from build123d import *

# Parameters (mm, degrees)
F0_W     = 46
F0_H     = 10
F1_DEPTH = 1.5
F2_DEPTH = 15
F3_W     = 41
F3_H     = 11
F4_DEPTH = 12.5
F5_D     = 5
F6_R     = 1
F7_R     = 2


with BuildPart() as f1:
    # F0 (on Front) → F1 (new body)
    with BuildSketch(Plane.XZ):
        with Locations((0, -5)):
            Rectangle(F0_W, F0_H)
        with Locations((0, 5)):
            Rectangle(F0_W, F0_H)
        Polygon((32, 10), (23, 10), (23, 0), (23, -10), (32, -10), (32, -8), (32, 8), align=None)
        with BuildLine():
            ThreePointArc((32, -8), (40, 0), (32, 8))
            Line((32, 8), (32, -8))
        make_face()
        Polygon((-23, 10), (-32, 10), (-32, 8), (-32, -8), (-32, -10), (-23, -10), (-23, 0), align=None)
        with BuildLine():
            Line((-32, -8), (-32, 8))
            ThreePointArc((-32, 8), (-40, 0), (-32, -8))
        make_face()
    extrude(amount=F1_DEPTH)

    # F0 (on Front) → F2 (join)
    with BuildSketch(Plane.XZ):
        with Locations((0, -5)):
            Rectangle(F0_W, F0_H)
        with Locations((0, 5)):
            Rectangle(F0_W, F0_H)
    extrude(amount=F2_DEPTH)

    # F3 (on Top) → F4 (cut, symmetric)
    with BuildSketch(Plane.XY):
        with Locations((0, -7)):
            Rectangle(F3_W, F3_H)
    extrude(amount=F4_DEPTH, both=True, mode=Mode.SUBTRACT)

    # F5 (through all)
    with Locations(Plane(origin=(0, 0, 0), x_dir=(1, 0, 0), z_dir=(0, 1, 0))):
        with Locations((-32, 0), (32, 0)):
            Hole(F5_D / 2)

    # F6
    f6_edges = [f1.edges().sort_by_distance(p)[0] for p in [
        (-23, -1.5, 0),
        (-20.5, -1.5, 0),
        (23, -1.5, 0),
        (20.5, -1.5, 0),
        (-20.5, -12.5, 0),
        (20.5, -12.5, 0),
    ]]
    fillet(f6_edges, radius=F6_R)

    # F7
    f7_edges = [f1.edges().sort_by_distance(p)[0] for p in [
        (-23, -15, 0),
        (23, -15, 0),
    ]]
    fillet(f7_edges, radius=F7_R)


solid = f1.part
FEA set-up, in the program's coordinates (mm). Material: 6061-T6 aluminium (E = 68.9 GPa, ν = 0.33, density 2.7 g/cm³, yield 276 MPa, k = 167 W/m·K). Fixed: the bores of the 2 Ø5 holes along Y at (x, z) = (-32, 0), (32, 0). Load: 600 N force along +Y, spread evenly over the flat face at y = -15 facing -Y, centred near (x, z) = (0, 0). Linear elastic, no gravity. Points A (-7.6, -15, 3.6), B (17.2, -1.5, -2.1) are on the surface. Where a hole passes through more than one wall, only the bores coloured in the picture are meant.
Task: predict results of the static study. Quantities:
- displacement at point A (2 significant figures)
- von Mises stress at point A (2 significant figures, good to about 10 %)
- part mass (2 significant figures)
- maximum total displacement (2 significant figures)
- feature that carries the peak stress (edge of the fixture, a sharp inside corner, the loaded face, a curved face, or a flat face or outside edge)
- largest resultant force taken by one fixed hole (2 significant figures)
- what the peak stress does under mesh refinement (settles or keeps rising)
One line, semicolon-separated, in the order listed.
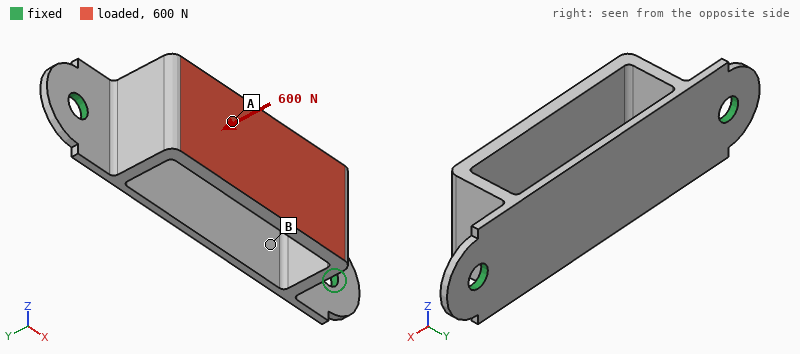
0.12 mm; 43 MPa; 15 g; 0.14 mm; edge of the fixture; 370 N; keeps rising
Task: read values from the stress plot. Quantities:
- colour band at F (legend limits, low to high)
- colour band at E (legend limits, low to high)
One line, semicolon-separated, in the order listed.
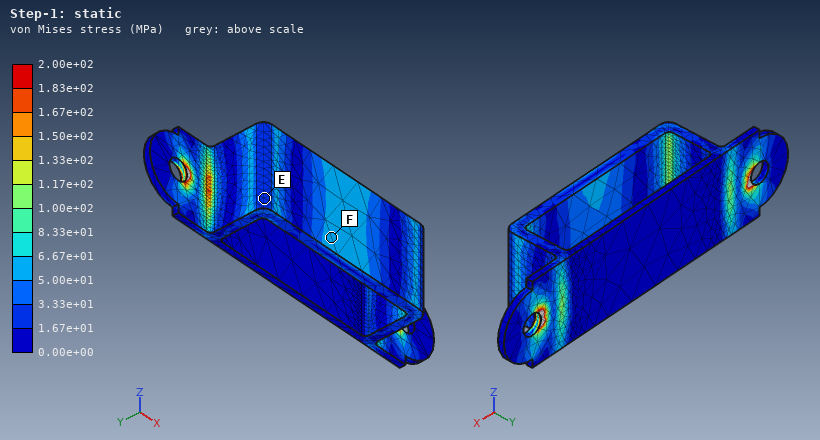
5.00e+01 to 6.67e+01 MPa; 1.67e+01 to 3.33e+01 MPa
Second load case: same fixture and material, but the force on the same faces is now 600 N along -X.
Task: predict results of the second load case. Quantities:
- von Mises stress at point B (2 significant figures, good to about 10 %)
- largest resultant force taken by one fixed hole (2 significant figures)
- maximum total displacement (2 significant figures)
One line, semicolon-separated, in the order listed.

56 MPa; 330 N; 0.13 mm
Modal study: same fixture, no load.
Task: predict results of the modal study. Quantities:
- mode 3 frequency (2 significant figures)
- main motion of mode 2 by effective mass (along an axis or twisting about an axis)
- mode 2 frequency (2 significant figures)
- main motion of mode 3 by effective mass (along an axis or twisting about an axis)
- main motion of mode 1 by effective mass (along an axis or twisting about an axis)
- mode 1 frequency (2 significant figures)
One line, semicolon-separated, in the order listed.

3800 Hz; along Y; 3500 Hz; along X; along Z; 2000 Hz
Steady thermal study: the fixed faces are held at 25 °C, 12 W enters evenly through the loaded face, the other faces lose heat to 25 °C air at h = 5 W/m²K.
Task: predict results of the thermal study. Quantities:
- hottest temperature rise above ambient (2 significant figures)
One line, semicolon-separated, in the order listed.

27 K
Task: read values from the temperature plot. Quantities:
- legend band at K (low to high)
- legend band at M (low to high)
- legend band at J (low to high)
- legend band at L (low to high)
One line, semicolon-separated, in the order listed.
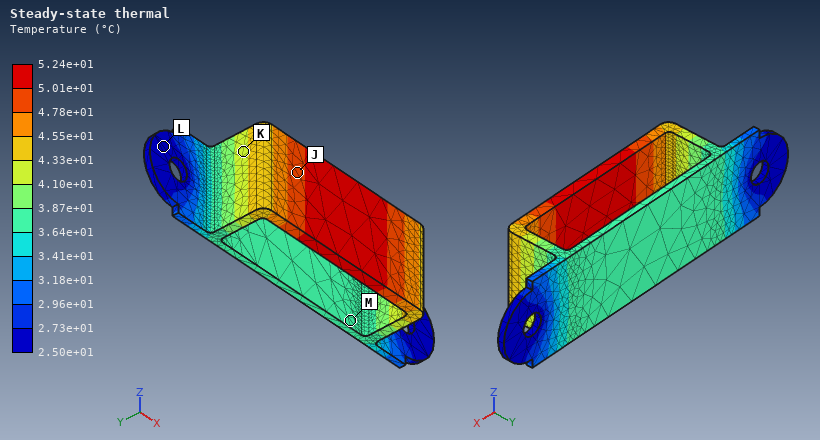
4.10e+01 to 4.33e+01 °C; 3.64e+01 to 3.87e+01 °C; 4.78e+01 to 5.01e+01 °C; 2.50e+01 to 2.73e+01 °C
